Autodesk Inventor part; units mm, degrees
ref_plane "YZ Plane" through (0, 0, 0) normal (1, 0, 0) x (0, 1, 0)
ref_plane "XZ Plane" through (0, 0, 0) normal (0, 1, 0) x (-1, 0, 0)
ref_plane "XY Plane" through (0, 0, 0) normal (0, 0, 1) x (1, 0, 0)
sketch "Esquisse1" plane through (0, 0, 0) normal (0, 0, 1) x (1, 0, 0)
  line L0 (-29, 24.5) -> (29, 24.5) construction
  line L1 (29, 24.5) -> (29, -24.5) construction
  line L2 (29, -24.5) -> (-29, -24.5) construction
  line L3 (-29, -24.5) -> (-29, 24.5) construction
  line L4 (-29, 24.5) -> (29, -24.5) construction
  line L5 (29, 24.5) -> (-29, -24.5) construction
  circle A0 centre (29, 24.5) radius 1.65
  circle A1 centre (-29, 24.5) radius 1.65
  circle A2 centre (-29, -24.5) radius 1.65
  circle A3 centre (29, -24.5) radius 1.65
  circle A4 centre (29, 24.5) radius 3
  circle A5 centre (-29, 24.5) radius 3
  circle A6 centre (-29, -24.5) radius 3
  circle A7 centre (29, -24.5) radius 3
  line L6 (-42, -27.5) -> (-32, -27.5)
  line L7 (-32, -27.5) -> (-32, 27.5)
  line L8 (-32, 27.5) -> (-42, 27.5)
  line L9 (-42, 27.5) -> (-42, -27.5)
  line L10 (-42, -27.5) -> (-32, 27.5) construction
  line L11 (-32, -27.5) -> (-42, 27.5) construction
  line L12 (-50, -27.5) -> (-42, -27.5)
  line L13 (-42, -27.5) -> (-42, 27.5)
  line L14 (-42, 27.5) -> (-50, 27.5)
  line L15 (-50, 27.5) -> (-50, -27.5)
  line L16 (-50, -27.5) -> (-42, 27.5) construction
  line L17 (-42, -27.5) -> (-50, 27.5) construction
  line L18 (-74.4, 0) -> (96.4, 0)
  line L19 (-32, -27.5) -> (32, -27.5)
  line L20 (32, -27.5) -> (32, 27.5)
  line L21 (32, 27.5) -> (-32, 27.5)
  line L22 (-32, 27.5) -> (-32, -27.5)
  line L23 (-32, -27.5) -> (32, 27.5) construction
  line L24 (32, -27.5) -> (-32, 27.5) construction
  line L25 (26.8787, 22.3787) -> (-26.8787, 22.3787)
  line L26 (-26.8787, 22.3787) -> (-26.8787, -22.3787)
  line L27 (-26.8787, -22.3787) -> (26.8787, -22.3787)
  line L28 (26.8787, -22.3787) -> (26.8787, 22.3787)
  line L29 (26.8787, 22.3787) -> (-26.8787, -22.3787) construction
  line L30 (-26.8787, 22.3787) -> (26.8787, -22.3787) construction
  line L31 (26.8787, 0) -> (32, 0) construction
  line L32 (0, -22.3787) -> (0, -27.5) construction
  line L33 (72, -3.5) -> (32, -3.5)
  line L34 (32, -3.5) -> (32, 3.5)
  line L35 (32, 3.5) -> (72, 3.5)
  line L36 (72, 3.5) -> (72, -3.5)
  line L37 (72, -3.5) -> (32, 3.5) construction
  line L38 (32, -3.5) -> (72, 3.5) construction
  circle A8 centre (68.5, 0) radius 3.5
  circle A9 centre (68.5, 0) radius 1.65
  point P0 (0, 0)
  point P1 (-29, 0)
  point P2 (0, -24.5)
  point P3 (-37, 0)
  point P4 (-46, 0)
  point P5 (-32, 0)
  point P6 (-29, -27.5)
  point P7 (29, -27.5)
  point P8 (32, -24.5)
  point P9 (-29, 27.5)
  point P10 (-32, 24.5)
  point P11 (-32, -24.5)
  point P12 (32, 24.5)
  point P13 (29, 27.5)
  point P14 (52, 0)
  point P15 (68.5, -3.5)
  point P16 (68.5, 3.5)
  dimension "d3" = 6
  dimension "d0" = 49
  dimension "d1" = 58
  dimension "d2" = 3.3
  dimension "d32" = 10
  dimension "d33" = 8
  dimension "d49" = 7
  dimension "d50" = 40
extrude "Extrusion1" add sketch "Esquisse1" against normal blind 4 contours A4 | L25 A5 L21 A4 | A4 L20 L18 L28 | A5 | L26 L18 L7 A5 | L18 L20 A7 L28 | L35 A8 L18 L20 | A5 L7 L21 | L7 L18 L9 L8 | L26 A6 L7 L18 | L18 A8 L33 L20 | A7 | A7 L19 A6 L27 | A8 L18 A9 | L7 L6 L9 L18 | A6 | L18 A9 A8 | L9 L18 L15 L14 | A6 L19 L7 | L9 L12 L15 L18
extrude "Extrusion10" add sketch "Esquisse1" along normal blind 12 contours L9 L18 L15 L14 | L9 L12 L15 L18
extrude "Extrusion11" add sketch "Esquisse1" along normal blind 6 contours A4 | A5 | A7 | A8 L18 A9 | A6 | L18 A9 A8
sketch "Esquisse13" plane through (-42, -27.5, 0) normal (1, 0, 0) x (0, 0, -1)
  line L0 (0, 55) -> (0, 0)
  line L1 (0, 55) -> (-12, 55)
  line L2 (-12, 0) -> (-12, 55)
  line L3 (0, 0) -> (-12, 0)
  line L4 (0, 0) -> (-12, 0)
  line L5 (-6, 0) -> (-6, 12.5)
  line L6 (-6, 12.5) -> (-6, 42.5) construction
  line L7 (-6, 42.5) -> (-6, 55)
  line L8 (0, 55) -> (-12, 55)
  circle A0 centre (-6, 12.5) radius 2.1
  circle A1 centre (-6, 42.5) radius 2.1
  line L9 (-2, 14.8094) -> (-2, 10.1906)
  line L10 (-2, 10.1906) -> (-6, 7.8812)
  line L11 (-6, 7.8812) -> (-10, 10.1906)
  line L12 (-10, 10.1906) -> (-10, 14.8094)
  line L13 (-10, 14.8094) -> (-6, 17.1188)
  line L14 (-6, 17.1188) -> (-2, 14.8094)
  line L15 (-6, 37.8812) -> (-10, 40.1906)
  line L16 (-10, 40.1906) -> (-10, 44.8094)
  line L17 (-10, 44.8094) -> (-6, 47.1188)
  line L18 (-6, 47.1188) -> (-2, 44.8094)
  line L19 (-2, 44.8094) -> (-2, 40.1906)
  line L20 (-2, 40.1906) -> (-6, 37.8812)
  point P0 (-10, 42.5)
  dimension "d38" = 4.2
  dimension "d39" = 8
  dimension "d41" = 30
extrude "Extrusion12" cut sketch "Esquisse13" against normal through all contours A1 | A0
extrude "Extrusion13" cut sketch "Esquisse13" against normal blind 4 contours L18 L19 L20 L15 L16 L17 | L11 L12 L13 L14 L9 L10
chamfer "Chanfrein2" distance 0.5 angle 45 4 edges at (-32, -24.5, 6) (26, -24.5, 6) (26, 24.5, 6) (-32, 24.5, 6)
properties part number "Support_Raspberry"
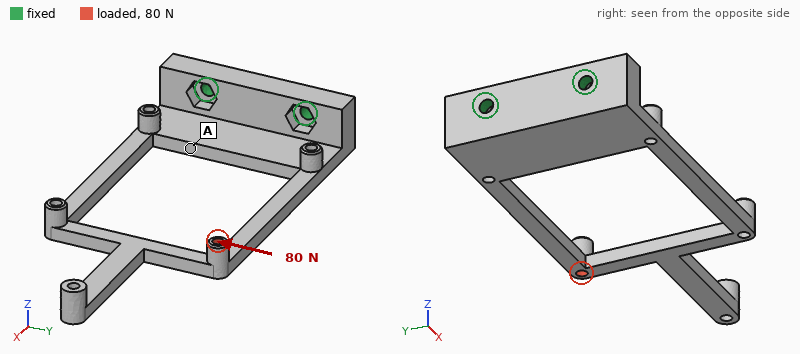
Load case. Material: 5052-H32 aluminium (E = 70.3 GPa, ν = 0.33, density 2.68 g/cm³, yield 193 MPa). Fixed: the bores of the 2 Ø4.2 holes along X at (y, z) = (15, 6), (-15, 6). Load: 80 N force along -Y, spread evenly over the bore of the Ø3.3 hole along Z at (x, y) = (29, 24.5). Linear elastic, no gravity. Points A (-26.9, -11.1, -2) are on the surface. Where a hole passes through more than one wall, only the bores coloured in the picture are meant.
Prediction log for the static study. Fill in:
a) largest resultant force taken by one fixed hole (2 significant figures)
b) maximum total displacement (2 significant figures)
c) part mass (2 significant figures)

190 N
0.40 mm
39 g
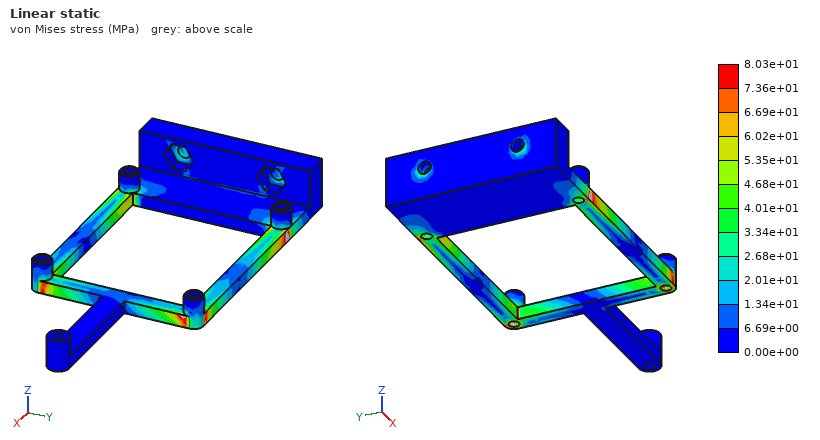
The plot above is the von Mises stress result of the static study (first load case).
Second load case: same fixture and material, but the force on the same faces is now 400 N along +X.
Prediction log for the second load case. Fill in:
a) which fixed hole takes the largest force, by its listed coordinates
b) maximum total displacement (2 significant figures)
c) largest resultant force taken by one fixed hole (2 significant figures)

(15, 6)
1.4 mm
500 N
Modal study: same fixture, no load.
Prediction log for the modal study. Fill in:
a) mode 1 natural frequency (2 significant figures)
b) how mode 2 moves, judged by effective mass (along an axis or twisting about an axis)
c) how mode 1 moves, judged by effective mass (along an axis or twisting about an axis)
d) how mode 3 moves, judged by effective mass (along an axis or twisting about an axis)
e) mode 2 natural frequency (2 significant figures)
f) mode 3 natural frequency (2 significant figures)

270 Hz
along Y
along Z
twisting about X
820 Hz
1100 Hz
